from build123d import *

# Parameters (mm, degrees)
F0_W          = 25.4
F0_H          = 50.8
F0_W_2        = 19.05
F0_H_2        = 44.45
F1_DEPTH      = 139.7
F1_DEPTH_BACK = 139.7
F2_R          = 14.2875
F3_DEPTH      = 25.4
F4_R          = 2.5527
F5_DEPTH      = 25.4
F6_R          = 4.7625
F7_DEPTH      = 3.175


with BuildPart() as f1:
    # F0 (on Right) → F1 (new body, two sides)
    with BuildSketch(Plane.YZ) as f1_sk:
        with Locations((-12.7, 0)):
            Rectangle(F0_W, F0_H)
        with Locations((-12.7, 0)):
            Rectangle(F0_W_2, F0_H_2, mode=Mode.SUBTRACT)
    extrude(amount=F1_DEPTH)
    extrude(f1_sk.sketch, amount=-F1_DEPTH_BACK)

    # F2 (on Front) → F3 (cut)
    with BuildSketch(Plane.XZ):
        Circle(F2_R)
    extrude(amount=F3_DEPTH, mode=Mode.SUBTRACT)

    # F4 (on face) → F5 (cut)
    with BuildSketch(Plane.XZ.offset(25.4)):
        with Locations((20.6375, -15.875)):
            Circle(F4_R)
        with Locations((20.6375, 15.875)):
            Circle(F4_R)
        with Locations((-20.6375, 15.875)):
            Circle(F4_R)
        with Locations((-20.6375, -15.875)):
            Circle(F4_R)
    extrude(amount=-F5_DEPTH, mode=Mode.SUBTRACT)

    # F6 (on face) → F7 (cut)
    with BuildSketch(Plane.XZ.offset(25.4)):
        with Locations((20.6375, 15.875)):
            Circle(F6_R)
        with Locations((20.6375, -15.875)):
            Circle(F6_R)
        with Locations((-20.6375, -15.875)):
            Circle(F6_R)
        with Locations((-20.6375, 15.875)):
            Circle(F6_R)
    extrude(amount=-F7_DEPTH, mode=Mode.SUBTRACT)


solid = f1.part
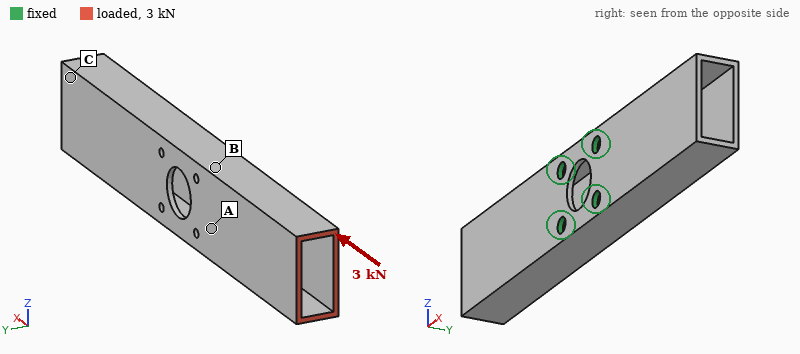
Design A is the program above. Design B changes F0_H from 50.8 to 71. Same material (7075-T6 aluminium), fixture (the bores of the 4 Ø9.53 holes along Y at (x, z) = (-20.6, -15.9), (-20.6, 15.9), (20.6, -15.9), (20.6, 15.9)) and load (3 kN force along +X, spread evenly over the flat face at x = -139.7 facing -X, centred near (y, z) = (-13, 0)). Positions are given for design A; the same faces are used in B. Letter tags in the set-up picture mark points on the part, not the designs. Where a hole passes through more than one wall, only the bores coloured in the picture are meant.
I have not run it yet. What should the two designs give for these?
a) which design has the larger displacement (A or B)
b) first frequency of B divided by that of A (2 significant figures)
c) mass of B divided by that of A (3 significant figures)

A
0.71
2.21
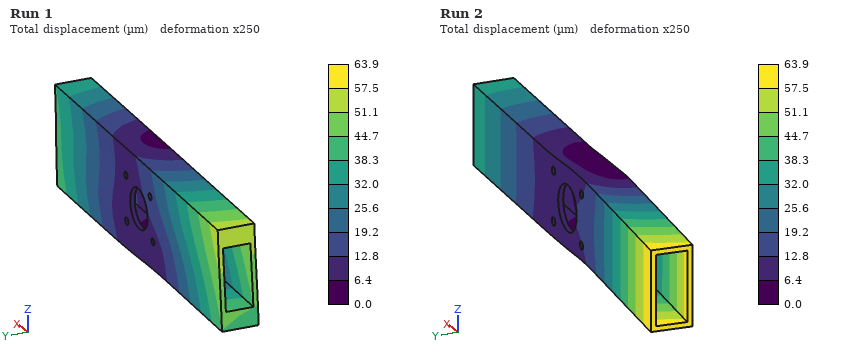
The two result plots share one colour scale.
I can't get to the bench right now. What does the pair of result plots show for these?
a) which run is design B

Run 1
